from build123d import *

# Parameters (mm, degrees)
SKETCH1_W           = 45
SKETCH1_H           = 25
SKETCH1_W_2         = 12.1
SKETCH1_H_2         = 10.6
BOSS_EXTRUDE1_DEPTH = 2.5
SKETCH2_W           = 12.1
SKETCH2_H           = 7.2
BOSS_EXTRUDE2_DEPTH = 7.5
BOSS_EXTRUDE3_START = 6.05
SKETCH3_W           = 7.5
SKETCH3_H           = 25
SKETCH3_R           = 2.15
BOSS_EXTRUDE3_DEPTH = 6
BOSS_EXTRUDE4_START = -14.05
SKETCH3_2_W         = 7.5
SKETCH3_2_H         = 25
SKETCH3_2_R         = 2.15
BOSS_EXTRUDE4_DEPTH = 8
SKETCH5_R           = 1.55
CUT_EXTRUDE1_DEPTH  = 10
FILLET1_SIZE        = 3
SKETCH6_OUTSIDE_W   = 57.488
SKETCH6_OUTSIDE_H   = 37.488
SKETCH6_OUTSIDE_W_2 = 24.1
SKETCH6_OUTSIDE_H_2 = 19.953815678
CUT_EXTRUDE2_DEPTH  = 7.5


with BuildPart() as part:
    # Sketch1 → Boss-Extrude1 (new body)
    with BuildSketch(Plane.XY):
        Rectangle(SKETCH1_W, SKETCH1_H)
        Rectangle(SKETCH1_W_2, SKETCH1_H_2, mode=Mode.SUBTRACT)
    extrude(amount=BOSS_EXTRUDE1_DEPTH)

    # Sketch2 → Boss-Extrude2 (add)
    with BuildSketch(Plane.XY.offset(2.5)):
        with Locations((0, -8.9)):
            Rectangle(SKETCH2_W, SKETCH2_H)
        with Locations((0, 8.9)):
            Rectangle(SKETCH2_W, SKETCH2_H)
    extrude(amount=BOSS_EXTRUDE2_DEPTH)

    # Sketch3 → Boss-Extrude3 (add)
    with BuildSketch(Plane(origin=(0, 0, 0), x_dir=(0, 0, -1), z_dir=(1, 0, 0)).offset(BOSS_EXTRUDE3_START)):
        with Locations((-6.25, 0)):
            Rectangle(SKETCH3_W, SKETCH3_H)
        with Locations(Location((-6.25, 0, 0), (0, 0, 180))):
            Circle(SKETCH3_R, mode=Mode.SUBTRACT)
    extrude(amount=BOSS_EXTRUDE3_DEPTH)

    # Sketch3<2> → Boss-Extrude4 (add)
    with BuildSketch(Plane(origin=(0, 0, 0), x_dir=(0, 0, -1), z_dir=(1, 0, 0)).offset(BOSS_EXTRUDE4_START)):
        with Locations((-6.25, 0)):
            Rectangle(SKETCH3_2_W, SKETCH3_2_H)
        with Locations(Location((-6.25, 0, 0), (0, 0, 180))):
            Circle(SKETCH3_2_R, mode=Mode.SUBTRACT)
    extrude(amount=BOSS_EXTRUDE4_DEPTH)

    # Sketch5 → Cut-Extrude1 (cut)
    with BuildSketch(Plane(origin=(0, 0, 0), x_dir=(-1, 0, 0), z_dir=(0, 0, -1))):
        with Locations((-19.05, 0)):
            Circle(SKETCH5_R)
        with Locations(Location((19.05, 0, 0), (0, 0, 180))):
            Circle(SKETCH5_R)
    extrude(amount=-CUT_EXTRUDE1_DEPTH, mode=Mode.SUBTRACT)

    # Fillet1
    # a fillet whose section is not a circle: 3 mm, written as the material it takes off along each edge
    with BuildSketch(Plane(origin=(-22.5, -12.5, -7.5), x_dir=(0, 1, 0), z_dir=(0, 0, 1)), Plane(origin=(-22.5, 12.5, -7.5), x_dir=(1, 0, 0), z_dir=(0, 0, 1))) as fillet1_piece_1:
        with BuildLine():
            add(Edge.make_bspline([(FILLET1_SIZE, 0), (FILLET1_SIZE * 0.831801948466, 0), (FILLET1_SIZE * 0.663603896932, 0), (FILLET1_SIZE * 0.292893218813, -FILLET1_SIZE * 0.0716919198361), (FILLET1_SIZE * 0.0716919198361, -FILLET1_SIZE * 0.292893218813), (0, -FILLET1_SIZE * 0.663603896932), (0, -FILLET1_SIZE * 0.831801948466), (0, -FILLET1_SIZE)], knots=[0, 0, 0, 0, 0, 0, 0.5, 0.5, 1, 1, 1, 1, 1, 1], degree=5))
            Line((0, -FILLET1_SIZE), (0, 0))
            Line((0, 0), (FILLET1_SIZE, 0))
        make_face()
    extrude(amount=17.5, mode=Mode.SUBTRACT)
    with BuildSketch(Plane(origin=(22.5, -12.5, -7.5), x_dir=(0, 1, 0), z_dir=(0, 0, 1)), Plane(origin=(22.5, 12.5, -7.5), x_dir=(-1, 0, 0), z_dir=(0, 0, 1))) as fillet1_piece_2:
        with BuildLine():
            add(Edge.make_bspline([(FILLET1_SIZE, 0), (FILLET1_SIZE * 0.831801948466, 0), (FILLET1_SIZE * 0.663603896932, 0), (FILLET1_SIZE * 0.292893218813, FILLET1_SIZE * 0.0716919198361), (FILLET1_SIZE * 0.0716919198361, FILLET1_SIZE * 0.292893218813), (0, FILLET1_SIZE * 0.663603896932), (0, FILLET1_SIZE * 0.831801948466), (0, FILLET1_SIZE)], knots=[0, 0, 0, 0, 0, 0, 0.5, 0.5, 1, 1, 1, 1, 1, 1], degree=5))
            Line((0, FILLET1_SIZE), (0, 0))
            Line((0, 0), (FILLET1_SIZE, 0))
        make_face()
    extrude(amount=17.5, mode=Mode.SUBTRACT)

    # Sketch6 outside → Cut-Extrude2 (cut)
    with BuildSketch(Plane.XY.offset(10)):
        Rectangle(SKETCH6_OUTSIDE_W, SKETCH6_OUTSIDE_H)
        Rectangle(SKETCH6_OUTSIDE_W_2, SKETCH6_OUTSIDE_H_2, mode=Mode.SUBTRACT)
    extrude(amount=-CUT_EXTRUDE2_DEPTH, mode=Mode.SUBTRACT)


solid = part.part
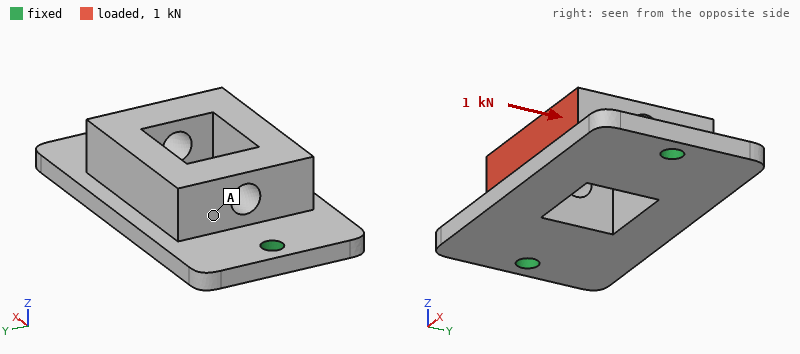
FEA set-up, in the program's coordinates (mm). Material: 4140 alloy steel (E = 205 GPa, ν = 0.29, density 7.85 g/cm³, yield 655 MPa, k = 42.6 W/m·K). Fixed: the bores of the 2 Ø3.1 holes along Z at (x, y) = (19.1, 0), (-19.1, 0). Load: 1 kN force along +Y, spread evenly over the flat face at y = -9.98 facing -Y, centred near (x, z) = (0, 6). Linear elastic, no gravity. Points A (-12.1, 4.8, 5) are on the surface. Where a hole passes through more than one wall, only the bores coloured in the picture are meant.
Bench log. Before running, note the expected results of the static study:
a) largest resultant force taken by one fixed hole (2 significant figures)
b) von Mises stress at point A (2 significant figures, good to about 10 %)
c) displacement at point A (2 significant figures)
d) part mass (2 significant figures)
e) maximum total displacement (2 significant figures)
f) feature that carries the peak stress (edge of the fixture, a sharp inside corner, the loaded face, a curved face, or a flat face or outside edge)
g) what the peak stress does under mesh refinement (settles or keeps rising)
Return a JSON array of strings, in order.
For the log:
["500 N", "21 MPa", "13 µm", "39 g", "31 µm", "edge of the fixture", "keeps rising"]
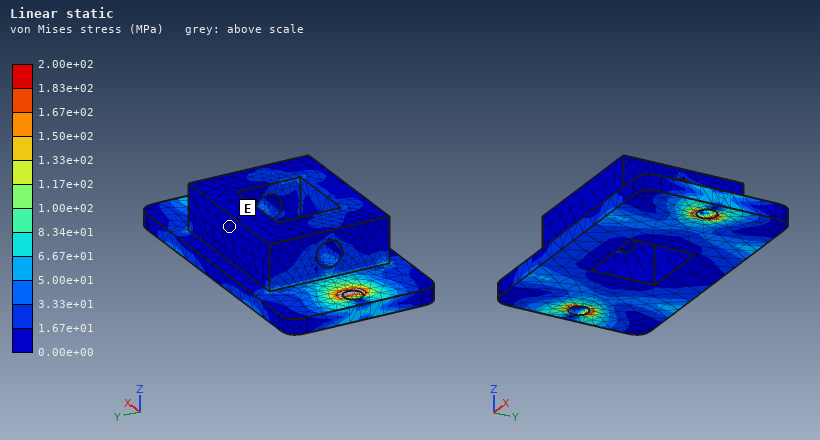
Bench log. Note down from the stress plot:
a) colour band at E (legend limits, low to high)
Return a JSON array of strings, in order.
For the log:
["0.00e+00 to 1.67e+01 MPa"]
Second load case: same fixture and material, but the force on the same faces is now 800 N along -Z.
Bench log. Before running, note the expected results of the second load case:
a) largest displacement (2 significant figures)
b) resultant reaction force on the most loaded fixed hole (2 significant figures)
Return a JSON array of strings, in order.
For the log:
["51 µm", "500 N"]
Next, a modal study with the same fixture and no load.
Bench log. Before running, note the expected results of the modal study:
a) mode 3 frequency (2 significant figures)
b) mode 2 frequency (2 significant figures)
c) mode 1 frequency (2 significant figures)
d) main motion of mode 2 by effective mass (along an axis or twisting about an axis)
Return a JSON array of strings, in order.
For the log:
["16 kHz", "9500 Hz", "5200 Hz", "along Z"]
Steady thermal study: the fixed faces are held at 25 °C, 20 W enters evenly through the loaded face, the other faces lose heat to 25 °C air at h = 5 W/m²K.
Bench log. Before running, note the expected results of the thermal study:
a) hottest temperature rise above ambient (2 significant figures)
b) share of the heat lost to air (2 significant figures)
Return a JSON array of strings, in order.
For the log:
["85 K", "3.5 %"]
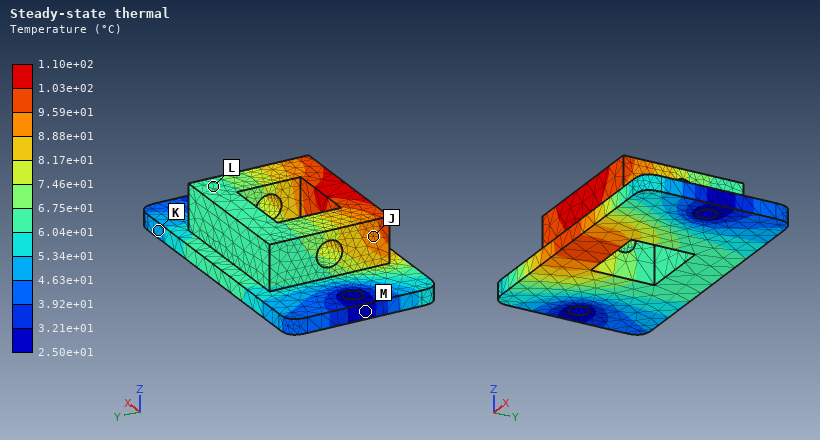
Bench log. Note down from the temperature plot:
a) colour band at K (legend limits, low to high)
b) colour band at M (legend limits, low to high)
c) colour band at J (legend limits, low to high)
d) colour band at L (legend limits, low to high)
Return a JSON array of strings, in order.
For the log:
["4.63e+01 to 5.34e+01 °C", "2.50e+01 to 3.21e+01 °C", "8.88e+01 to 9.59e+01 °C", "6.04e+01 to 6.75e+01 °C"]
